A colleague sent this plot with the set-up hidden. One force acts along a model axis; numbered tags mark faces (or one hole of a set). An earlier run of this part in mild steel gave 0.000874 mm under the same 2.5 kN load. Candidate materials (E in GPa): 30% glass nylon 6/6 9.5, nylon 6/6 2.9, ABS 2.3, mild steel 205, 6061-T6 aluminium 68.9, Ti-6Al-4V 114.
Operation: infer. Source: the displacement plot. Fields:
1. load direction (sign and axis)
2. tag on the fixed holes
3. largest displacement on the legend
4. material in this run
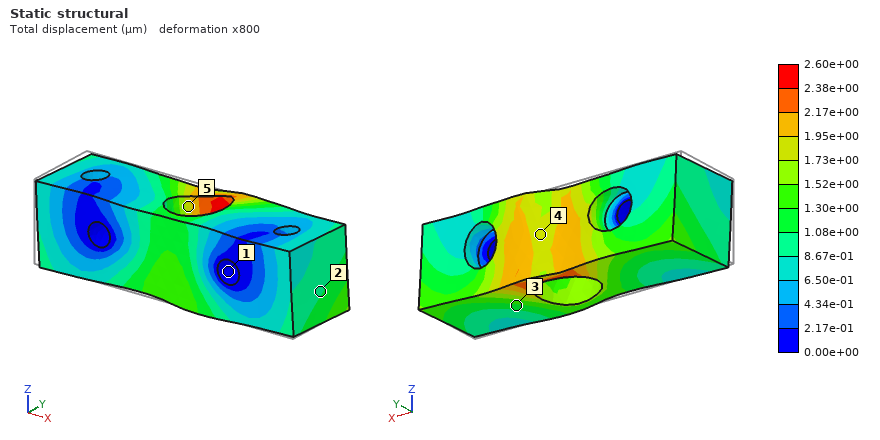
+X
1
2.60e+00 µm
6061-T6 aluminium
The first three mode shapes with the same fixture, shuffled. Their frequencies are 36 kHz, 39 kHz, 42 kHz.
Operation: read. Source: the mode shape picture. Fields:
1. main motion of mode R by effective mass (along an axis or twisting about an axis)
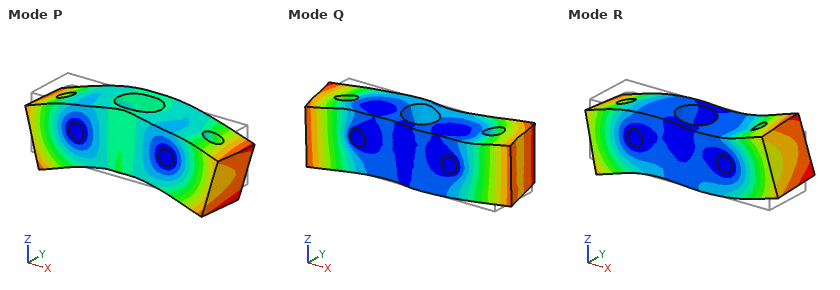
twisting about Y
